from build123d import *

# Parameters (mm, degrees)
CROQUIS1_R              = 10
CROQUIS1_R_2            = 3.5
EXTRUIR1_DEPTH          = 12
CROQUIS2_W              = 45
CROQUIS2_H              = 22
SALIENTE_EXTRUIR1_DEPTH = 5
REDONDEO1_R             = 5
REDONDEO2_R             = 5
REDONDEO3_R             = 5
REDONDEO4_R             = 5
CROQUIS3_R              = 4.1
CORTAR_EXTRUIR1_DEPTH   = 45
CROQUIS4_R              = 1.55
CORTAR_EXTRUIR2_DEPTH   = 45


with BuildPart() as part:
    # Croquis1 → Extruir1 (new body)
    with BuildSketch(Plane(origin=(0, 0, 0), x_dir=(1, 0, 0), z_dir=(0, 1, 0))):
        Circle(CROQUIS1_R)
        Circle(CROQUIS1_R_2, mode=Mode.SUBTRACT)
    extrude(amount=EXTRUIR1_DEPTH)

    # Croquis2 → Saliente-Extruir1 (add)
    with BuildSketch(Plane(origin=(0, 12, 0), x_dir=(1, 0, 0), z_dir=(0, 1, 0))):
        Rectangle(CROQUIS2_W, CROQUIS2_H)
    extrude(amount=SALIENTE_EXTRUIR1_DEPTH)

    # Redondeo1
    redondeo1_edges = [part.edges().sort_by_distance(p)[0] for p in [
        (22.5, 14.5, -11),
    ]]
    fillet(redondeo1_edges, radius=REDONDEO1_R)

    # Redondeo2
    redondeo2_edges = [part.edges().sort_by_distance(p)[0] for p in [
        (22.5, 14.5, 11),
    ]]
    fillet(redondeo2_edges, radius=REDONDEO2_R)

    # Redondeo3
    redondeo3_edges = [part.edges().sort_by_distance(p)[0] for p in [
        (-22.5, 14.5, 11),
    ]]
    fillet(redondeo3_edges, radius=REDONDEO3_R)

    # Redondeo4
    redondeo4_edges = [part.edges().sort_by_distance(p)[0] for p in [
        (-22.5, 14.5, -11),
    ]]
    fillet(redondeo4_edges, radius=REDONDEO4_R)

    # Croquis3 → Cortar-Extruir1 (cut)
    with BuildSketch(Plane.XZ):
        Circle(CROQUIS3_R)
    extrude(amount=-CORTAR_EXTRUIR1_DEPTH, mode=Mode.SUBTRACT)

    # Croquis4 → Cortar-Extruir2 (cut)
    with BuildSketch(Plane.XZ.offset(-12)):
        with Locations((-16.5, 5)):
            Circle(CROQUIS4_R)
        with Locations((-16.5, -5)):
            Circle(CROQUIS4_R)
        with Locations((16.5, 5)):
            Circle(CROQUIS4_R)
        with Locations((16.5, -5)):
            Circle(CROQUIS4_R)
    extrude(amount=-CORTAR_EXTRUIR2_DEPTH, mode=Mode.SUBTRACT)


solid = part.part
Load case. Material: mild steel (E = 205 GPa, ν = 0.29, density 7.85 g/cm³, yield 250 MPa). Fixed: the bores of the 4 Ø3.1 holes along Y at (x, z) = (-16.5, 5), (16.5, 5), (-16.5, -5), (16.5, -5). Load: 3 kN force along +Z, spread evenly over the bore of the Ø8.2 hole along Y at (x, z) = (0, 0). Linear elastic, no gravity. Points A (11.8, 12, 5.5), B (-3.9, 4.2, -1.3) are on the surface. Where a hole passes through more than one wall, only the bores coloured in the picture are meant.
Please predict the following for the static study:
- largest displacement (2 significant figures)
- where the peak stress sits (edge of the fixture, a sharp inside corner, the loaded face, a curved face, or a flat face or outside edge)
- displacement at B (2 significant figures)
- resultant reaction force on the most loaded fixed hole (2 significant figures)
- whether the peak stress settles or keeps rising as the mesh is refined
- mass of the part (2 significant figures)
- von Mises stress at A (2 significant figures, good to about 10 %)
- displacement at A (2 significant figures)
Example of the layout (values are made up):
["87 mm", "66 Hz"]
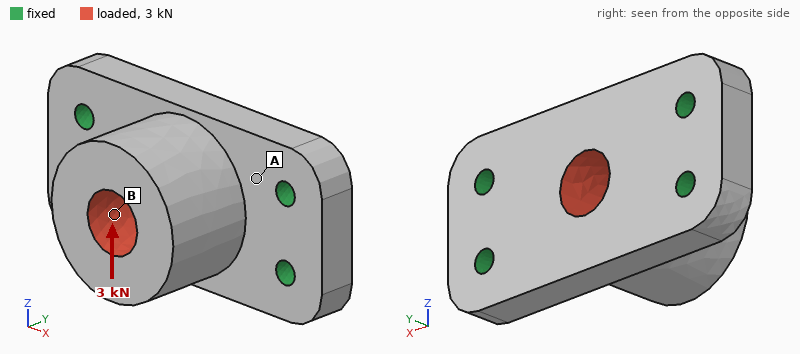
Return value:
["15 µm", "edge of the fixture", "10 µm", "1.2 kN", "keeps rising", "59 g", "62 MPa", "2.4 µm"]
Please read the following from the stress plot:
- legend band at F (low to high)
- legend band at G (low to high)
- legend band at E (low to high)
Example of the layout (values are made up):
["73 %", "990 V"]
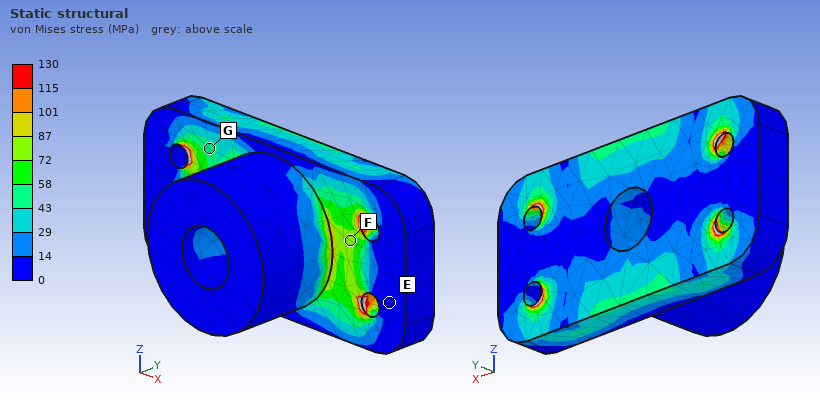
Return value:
["72 to 87 MPa", "43 to 58 MPa", "0 to 14 MPa"]
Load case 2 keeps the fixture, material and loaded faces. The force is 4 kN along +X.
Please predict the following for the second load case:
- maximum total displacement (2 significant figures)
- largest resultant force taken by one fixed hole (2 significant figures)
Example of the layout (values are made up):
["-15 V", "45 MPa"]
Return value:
["5.9 µm", "1.1 kN"]
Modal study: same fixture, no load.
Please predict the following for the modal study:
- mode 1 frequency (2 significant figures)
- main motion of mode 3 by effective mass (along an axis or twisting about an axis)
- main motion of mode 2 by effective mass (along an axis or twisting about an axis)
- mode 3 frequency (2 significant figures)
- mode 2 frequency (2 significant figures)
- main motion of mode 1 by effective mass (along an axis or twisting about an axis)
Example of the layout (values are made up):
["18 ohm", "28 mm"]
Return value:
["13 kHz", "along X", "along Y", "25 kHz", "19 kHz", "along Z"]
